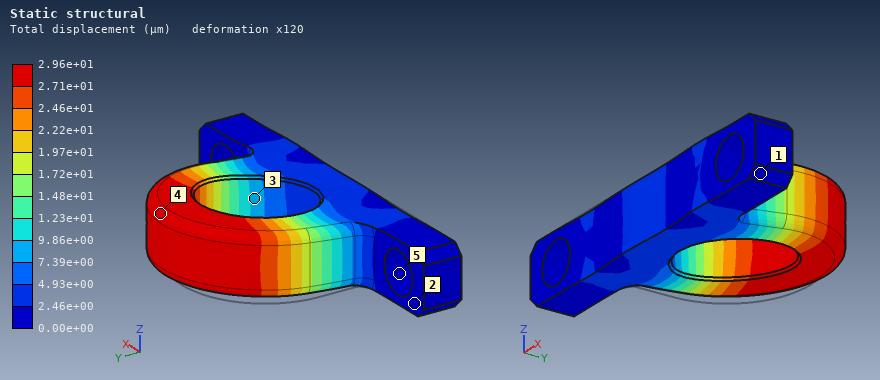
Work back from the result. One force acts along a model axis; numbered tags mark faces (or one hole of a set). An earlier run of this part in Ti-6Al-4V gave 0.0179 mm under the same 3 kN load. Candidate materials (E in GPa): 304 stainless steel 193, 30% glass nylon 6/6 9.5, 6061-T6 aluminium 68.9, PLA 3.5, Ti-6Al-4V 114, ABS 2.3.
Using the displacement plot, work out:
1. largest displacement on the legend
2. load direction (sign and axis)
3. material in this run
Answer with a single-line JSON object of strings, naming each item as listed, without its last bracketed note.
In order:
{"largest displacement on the legend": "2.96e+01 µm", "load direction": "+X", "material in this run": "6061-T6 aluminium"}
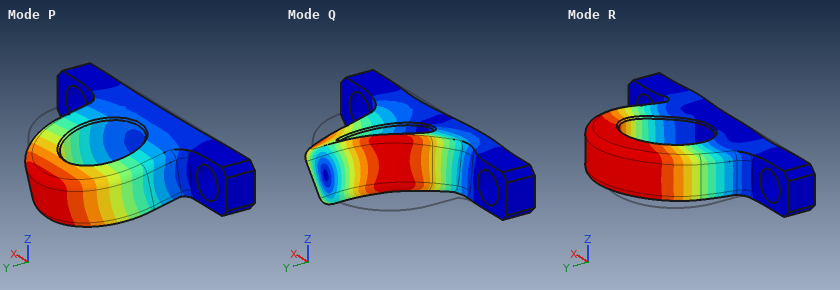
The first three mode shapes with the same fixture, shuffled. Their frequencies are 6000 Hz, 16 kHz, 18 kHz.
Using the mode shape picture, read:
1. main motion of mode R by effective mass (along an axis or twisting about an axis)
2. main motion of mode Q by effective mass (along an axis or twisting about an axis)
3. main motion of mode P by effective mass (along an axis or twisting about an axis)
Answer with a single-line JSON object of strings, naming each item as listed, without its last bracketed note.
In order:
{"main motion of mode R by effective mass": "along X", "main motion of mode Q by effective mass": "twisting about Y", "main motion of mode P by effective mass": "along Z"}
